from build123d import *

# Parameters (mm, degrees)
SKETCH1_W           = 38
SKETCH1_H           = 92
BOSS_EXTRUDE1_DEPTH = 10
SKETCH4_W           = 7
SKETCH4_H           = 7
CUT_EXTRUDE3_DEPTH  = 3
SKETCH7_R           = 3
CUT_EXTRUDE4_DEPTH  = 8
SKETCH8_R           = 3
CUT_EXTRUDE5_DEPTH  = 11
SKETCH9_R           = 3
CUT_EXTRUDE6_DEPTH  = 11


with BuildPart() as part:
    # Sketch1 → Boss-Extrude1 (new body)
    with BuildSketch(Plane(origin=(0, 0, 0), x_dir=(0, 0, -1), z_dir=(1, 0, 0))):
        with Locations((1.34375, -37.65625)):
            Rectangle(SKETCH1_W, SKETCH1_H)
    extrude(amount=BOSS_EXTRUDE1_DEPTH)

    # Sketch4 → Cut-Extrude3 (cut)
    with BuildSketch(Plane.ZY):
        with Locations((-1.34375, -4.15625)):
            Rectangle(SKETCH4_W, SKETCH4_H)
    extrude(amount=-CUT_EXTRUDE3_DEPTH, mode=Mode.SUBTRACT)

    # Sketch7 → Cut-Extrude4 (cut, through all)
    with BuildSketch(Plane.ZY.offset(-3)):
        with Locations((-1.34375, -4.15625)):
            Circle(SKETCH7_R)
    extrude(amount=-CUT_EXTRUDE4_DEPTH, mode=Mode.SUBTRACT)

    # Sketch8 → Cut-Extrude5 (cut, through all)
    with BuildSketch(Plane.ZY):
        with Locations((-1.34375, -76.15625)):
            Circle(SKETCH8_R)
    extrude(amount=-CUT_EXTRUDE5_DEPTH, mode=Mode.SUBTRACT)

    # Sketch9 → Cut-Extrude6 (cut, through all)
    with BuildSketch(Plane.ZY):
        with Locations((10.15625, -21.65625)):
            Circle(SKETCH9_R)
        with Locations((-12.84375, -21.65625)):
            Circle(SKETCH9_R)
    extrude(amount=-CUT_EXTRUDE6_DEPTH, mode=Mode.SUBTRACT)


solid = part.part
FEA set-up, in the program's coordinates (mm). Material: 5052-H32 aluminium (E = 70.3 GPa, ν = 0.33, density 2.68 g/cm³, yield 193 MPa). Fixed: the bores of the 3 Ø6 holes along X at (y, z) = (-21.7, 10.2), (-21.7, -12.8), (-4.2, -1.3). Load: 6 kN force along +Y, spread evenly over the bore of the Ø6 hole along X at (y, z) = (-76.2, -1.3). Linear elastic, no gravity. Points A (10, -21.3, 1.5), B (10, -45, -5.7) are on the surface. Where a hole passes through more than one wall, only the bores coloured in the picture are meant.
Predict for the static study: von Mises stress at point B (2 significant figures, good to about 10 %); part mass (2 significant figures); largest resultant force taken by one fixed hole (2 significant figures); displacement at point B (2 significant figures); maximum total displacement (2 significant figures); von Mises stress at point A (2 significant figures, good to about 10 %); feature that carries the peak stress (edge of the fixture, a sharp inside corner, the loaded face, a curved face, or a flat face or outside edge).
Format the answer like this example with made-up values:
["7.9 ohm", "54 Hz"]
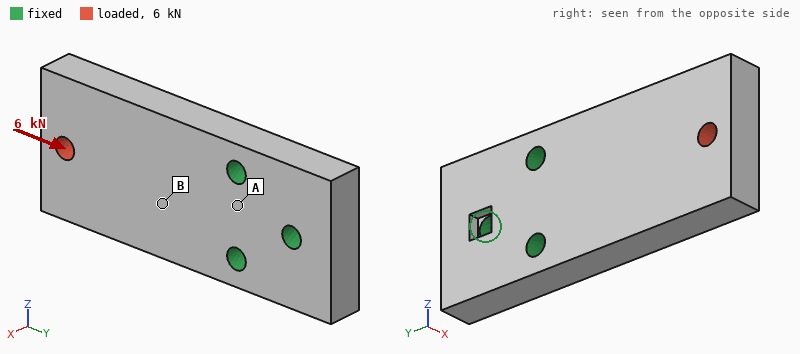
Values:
["17 MPa", "90 g", "2.8 kN", "5.4 µm", "20 µm", "7.0 MPa", "the loaded face"]
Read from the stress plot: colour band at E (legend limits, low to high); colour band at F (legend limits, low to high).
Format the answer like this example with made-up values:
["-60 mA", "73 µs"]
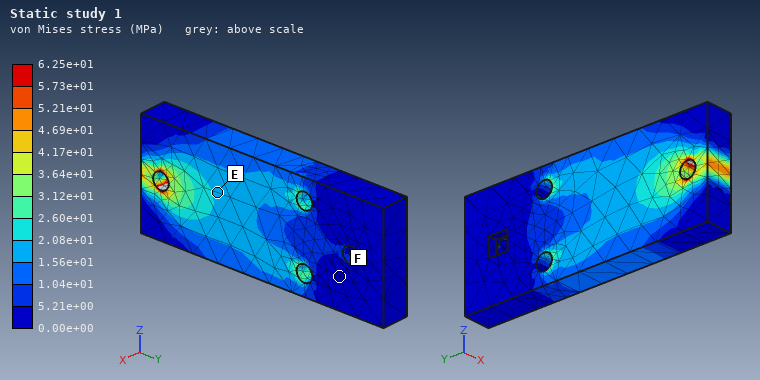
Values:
["1.56e+01 to 2.08e+01 MPa", "0.00e+00 to 5.21e+00 MPa"]
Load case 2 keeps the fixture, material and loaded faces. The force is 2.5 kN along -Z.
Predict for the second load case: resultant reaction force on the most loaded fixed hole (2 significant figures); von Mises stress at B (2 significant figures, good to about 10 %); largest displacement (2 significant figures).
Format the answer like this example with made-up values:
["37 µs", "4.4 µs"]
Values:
["5.1 kN", "18 MPa", "71 µm"]
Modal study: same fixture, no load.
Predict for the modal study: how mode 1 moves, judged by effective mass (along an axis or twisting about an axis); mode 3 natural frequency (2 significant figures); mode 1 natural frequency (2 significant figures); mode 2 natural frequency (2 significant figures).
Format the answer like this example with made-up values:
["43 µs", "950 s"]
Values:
["along X", "6800 Hz", "2200 Hz", "6600 Hz"]
